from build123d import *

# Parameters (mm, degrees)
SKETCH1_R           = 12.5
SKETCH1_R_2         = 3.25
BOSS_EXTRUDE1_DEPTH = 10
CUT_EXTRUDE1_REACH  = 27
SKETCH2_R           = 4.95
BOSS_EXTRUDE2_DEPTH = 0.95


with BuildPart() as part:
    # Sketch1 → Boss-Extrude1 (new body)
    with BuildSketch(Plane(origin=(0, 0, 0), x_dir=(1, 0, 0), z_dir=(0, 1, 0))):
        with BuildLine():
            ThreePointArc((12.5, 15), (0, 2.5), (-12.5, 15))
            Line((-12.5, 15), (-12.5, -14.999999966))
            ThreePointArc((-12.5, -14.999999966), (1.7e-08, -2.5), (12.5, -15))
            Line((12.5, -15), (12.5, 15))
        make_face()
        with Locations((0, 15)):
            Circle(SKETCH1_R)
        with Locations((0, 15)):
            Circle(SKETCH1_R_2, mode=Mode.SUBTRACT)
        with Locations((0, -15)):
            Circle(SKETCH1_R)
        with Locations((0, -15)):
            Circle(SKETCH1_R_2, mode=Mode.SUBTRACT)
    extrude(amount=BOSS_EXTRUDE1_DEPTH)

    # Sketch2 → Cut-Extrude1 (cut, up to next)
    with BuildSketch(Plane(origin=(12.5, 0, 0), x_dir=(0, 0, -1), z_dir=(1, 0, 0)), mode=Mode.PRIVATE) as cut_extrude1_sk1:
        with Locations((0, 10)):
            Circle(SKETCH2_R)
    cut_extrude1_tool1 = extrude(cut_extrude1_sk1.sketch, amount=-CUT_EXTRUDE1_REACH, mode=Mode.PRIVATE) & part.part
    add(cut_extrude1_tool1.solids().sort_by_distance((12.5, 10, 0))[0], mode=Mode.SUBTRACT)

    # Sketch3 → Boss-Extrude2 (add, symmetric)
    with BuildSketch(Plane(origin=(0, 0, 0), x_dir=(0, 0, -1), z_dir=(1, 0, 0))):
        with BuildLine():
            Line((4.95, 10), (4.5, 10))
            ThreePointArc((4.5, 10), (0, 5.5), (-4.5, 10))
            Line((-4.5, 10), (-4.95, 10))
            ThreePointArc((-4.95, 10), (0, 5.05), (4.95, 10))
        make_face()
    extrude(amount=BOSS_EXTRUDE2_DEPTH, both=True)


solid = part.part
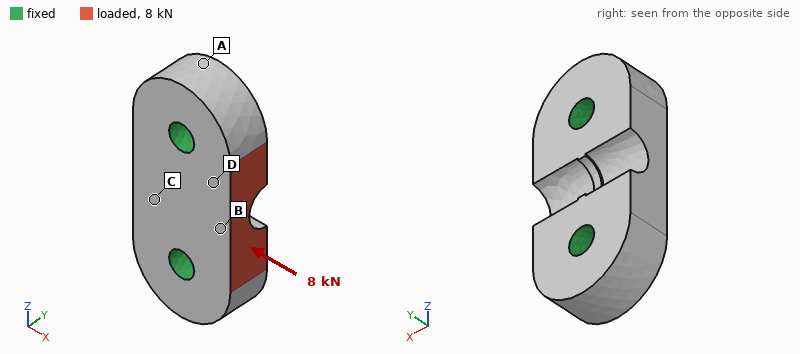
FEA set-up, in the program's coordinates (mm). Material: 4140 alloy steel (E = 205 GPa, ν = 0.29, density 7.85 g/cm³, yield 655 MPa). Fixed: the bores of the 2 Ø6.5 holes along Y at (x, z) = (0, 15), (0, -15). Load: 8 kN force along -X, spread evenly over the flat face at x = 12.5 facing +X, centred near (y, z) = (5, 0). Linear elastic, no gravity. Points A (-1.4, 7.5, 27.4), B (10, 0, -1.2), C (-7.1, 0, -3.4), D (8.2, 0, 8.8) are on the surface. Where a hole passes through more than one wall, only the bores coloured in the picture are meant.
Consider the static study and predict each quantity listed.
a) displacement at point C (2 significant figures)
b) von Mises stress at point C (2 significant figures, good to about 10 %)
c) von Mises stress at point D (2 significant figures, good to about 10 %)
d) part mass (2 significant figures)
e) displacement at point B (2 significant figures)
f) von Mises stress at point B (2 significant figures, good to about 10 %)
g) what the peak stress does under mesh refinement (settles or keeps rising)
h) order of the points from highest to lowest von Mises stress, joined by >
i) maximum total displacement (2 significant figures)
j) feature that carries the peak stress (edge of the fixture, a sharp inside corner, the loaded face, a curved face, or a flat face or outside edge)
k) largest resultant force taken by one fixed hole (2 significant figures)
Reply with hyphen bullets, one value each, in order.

- 1.9 µm
- 15 MPa
- 33 MPa
- 85 g
- 3.6 µm
- 24 MPa
- keeps rising
- D > B > C > A
- 4.0 µm
- edge of the fixture
- 4.1 kN
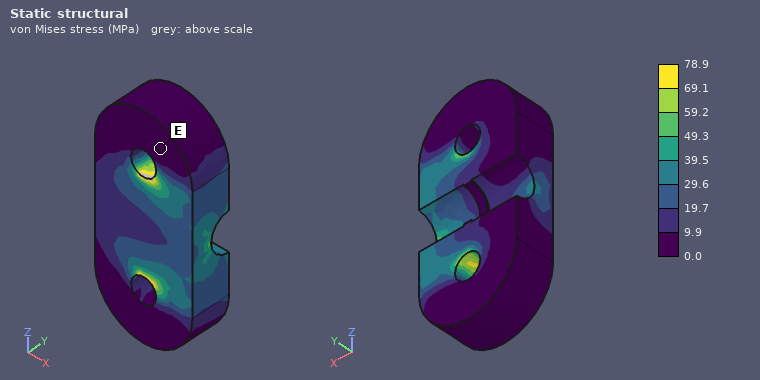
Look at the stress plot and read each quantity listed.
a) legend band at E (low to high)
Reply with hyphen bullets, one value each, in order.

- 0.0 to 9.9 MPa
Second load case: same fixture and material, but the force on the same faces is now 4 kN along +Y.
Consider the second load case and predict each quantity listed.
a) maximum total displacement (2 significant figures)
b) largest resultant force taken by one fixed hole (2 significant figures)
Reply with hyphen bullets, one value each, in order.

- 10 µm
- 2.0 kN
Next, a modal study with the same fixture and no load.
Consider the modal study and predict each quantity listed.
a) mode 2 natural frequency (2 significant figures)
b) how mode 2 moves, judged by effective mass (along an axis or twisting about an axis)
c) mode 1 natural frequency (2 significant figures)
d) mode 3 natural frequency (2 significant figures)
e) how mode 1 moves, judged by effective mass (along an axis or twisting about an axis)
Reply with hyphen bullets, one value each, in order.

- 36 kHz
- along Y
- 35 kHz
- 42 kHz
- twisting about Z
